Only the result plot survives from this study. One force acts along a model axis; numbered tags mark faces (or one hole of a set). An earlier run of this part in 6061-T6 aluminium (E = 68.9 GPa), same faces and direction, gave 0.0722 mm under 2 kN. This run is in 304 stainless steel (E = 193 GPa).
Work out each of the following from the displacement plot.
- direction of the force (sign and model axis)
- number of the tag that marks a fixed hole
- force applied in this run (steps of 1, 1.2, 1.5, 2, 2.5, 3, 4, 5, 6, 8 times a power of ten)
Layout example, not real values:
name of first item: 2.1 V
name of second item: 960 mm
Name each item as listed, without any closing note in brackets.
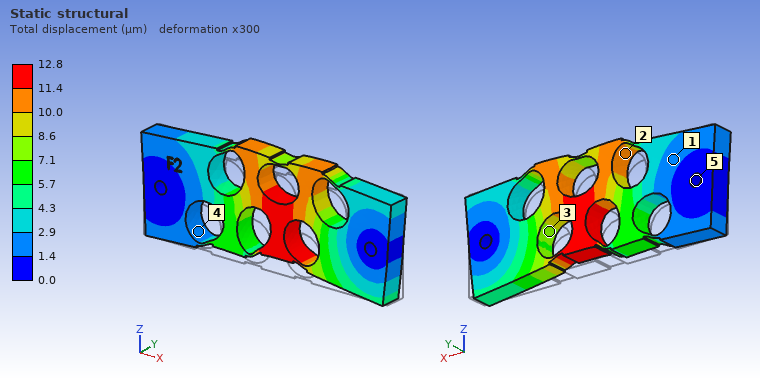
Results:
direction of the force: +Z
number of the tag that marks a fixed hole: 5
force applied in this run: 1 kN
